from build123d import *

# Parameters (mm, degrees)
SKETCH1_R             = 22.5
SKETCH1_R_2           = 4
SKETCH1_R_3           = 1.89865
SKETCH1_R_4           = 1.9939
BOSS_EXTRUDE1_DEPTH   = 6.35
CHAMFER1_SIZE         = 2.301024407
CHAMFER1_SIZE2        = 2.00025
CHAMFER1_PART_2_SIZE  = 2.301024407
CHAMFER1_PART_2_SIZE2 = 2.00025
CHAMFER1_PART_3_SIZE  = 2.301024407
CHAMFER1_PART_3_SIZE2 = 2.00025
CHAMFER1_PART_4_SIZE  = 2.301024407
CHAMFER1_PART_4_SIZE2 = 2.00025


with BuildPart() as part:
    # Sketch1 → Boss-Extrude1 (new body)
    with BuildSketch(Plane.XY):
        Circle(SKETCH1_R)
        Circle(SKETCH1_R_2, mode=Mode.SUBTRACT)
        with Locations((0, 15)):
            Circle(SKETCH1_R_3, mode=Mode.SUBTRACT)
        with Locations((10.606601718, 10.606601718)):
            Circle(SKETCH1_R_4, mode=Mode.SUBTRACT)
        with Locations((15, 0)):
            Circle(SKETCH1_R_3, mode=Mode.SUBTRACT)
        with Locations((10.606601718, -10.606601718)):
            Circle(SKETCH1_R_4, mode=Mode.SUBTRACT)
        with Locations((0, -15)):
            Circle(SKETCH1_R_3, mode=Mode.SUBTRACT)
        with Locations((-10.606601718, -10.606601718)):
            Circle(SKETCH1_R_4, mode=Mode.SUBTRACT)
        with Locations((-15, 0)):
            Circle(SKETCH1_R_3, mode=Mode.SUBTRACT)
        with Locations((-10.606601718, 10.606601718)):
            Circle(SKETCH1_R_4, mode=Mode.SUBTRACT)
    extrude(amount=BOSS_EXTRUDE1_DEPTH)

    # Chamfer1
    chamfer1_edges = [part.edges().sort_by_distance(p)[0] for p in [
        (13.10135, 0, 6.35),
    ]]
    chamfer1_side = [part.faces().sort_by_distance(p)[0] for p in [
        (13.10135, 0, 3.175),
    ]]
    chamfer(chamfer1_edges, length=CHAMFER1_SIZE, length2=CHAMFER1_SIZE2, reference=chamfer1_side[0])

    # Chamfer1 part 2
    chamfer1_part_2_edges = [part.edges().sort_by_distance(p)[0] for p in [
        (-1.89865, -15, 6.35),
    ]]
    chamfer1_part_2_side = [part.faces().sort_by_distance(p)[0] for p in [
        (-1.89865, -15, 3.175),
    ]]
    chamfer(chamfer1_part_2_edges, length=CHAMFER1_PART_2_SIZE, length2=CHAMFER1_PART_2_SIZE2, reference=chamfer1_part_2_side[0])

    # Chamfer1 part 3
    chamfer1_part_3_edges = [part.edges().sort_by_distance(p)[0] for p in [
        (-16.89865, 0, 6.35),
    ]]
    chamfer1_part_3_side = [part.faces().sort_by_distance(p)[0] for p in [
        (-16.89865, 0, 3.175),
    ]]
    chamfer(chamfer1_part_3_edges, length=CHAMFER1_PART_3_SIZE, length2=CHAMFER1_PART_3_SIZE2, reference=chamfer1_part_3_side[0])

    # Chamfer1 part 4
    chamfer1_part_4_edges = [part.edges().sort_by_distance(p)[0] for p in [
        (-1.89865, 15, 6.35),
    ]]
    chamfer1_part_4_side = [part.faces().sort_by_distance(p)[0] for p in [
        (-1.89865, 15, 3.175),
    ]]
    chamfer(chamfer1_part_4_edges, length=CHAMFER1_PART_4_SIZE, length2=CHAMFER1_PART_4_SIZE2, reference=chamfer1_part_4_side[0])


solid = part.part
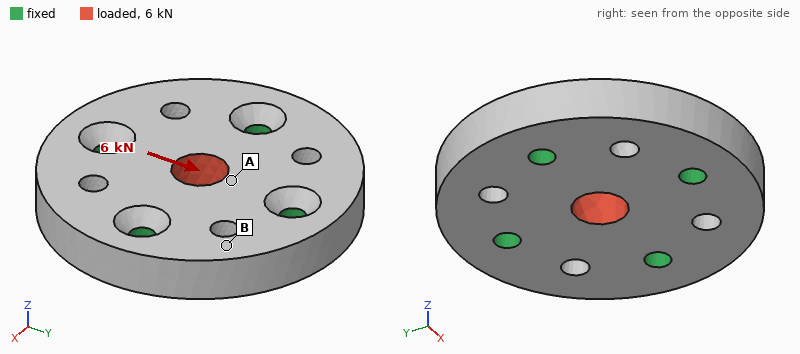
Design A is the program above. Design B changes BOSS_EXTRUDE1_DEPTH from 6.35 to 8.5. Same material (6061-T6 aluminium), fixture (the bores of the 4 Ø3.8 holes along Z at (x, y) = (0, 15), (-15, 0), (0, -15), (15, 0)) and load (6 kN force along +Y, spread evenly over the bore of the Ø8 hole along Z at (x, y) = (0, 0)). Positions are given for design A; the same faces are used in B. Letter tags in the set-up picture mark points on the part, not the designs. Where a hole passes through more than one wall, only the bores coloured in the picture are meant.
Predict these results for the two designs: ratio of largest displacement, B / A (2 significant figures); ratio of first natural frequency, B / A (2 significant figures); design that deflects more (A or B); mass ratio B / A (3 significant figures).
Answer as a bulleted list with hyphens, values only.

- 0.73
- 1.3
- A
- 1.34
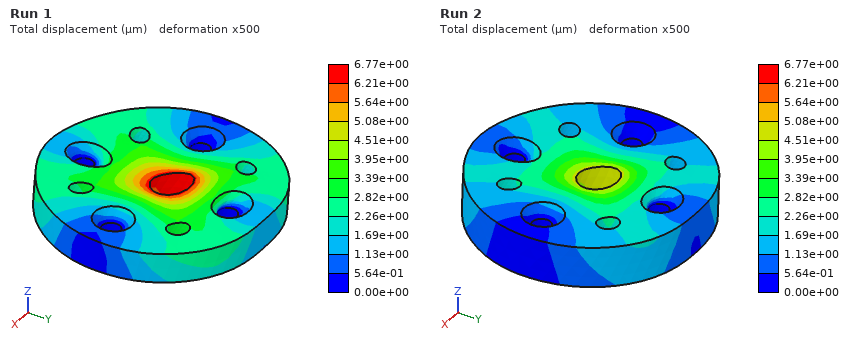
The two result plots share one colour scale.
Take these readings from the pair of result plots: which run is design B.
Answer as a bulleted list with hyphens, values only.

- Run 2
